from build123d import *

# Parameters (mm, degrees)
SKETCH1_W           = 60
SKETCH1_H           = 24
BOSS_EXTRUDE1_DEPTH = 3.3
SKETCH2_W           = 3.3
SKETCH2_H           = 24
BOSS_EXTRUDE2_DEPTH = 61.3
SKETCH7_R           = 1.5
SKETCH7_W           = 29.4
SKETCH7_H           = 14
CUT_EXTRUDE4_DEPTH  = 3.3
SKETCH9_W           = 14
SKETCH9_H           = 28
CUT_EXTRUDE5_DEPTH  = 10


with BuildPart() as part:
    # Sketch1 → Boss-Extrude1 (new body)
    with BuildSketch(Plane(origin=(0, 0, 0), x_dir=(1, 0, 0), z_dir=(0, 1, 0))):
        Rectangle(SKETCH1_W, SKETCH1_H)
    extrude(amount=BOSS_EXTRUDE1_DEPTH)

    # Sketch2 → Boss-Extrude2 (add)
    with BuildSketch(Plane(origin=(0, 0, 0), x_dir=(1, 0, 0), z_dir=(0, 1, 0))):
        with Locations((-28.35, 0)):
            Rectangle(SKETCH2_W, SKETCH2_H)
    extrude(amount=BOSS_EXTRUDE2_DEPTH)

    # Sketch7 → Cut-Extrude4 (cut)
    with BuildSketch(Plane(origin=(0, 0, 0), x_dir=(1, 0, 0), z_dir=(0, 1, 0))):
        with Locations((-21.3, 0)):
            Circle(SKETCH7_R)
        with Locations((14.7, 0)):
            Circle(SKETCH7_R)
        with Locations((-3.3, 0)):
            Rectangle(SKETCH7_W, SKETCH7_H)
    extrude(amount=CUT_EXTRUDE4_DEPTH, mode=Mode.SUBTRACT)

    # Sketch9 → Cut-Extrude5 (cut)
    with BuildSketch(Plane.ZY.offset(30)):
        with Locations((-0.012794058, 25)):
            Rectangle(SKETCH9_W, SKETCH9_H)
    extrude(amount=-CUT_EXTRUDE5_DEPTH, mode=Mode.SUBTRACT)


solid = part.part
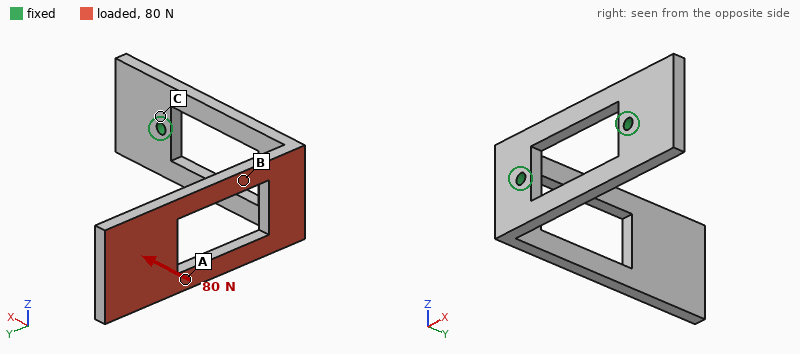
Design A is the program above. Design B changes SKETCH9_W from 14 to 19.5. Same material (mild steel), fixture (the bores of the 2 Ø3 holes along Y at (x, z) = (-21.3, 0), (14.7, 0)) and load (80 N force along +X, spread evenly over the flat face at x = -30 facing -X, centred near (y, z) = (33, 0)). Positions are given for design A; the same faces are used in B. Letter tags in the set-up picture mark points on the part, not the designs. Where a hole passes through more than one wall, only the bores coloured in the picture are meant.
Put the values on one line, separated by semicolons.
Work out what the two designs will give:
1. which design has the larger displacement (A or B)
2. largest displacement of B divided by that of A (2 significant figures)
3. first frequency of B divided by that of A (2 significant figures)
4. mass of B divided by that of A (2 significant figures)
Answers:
B; 1.9; 0.77; 0.92
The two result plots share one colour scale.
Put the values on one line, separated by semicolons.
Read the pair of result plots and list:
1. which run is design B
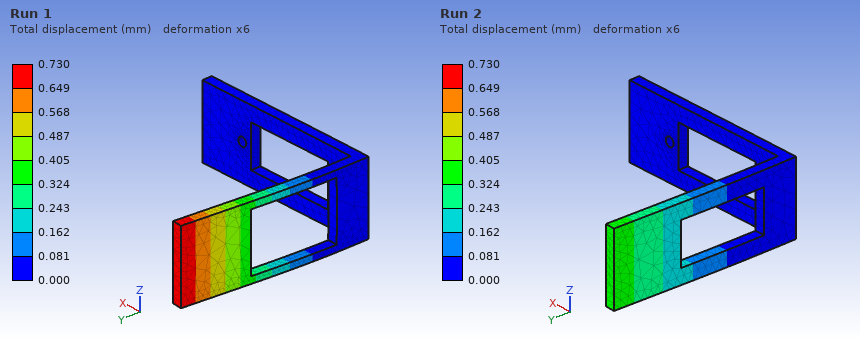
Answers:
Run 1
